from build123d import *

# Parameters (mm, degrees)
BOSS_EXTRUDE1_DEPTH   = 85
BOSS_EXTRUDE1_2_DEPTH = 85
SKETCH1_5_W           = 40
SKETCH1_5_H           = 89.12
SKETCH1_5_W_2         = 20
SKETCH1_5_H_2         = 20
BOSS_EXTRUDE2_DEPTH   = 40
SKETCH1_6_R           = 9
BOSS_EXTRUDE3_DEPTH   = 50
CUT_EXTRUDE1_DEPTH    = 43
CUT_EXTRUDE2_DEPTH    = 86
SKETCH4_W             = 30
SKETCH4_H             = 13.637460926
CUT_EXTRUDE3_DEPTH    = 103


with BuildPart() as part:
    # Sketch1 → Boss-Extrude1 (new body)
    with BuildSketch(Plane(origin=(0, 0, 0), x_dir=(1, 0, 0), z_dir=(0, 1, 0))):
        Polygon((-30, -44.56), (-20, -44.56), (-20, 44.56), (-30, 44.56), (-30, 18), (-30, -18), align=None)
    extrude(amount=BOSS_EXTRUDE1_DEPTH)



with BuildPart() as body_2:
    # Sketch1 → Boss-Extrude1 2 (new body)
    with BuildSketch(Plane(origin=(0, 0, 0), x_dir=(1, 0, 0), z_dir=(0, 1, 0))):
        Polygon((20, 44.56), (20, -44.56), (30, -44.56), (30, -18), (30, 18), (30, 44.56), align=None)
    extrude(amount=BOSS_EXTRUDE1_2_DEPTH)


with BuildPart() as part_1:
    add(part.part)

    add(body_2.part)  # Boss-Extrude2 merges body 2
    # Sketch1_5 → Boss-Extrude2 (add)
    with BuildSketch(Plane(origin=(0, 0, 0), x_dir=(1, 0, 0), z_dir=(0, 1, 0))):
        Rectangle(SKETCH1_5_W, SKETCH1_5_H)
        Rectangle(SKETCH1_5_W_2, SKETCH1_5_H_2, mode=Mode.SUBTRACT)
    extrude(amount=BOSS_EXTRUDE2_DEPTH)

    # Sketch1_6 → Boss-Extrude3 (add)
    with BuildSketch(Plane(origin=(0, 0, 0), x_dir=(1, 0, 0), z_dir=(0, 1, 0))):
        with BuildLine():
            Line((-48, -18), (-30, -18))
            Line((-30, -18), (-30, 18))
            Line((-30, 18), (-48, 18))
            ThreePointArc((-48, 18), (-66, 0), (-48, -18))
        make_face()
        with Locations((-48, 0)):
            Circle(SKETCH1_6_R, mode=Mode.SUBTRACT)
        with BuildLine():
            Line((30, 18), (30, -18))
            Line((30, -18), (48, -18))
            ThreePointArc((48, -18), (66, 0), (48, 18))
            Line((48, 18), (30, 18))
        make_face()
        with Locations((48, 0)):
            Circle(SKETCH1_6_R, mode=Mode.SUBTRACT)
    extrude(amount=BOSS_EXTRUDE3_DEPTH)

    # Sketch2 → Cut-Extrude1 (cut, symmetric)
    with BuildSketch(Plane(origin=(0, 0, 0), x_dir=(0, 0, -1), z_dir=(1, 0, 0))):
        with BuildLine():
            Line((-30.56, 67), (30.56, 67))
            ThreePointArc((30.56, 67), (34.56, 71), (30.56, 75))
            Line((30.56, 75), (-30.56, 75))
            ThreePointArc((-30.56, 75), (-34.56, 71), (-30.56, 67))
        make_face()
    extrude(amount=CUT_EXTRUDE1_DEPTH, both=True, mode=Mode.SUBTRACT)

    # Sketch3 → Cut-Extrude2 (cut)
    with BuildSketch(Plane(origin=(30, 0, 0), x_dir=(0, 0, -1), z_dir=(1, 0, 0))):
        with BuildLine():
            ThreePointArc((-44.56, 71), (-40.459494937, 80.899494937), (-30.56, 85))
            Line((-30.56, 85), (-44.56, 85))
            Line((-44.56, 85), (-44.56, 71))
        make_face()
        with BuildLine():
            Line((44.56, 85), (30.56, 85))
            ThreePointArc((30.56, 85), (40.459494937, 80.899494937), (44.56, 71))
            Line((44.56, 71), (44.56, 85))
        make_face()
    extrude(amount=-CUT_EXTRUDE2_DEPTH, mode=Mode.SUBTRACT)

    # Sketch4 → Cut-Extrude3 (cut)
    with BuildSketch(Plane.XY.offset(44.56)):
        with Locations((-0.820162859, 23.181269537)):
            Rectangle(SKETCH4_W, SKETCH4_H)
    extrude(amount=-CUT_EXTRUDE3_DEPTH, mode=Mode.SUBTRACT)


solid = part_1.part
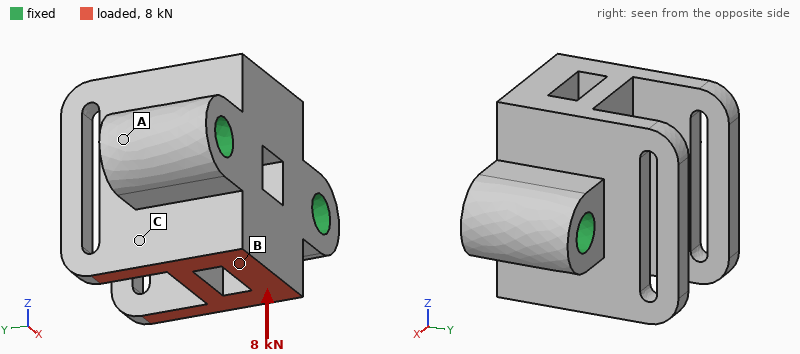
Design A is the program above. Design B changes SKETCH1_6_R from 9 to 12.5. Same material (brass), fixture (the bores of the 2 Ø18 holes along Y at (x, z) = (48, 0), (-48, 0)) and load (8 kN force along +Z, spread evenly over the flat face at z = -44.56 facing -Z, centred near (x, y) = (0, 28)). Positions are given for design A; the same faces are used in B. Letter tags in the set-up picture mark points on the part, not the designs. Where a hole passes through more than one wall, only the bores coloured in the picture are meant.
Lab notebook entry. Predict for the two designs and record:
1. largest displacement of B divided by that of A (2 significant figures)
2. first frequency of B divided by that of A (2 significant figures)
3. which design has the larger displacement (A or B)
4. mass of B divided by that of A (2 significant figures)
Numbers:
0.84
1.0
A
0.93
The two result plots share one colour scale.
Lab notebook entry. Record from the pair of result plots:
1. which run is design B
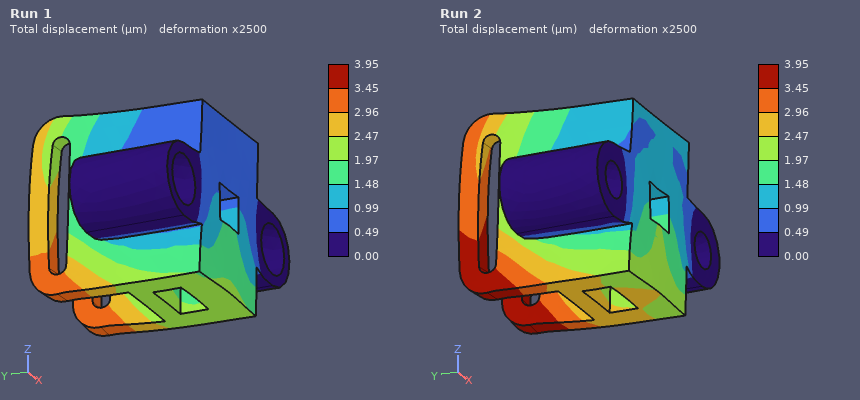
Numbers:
Run 1
